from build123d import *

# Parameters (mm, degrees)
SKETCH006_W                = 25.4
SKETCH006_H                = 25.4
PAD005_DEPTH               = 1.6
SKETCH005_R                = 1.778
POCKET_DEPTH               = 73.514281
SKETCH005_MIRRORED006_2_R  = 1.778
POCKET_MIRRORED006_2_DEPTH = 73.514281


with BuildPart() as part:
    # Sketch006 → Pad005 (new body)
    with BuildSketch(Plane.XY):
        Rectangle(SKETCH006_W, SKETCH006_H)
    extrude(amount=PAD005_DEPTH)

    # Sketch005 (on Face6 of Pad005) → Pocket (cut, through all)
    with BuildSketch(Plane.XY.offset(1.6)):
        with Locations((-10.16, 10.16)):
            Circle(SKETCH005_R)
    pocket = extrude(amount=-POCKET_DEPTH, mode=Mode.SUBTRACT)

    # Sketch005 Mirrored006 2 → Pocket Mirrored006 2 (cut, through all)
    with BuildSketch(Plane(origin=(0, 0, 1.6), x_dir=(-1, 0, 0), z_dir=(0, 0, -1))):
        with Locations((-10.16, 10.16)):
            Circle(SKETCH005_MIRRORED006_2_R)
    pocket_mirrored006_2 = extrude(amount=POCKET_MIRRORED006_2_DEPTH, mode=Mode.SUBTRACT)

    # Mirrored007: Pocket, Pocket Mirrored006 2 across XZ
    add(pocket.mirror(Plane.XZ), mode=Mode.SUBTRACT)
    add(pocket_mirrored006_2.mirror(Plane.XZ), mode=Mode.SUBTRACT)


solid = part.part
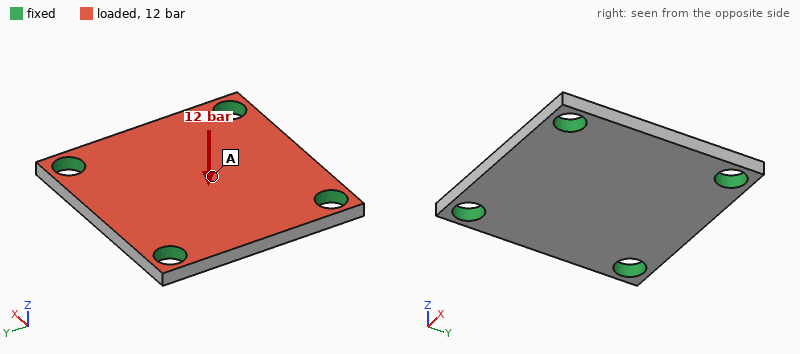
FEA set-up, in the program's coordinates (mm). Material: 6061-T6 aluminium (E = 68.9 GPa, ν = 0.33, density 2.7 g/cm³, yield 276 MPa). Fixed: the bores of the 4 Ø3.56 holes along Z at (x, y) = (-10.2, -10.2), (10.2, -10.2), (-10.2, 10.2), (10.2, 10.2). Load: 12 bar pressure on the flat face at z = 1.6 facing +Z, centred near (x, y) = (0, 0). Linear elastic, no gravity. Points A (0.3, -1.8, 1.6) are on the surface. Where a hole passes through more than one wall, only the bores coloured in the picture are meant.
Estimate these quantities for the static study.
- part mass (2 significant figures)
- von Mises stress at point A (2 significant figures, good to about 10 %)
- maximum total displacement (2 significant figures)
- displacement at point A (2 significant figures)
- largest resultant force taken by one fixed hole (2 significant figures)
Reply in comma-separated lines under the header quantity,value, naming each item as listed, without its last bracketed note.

quantity,value
part mass,2.6 g
von Mises stress at point A,46 MPa
maximum total displacement,37 µm
displacement at point A,36 µm
largest resultant force taken by one fixed hole,180 N
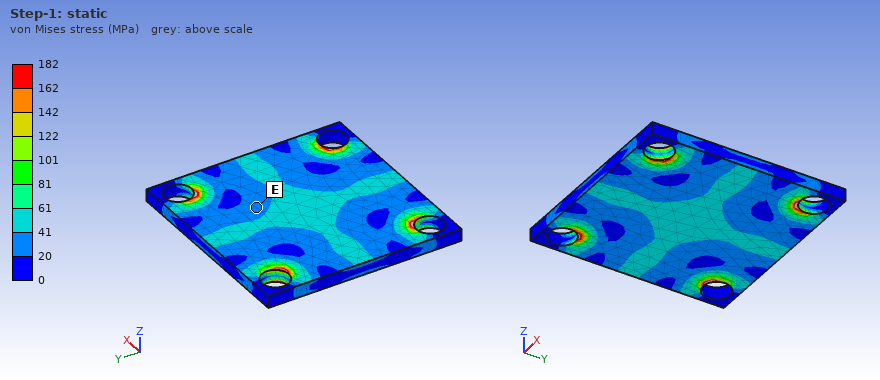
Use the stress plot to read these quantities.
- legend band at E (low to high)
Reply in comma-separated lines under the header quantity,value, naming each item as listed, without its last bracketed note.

quantity,value
legend band at E,20 to 41 MPa
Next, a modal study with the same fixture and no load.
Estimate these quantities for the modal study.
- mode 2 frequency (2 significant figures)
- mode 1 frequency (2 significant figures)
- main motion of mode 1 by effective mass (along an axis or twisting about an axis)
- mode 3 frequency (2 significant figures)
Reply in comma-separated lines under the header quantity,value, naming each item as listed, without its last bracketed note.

quantity,value
mode 2 frequency,27 kHz
mode 1 frequency,17 kHz
main motion of mode 1 by effective mass,along Z
mode 3 frequency,27 kHz
